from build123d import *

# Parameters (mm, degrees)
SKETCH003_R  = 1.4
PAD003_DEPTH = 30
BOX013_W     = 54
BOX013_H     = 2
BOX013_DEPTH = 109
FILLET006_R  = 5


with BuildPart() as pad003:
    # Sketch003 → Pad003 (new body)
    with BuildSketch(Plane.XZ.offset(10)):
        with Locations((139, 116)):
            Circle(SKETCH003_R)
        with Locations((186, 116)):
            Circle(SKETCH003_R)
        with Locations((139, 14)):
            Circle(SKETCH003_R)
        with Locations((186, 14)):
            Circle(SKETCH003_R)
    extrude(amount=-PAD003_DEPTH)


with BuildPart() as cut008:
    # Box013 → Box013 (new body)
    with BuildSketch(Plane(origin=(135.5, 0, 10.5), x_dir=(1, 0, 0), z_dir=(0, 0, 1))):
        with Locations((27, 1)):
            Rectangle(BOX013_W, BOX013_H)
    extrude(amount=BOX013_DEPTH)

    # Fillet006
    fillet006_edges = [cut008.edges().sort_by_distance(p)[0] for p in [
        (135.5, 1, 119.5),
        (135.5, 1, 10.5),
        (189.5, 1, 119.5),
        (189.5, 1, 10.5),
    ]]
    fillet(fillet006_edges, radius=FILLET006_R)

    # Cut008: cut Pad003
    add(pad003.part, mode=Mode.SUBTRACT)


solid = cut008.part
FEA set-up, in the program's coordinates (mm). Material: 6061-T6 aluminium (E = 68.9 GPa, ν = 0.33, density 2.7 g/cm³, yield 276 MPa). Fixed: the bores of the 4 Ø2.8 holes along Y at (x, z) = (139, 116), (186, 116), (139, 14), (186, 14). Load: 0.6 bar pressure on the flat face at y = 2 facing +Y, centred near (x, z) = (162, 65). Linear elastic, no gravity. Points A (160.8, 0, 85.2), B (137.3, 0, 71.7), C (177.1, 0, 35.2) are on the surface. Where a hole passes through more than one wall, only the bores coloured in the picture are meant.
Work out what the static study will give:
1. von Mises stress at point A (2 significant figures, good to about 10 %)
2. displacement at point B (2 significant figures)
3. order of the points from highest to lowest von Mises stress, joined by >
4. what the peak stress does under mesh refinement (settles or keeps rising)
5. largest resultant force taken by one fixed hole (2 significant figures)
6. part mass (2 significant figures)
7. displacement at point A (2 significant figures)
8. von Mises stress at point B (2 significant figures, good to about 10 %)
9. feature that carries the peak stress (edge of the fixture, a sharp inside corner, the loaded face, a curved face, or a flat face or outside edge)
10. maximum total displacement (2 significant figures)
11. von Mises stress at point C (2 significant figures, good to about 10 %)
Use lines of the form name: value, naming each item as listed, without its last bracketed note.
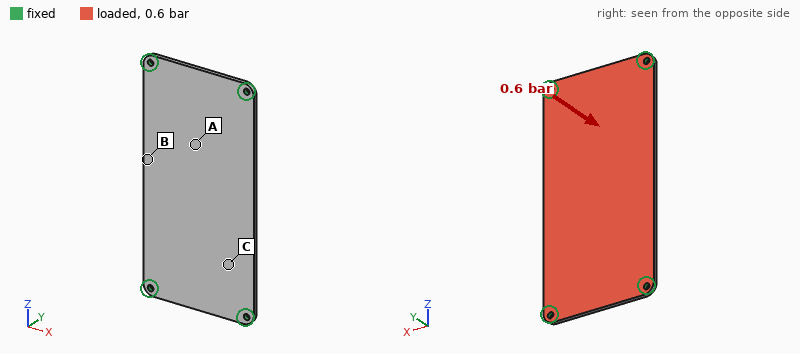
von Mises stress at point A: 25 MPa
displacement at point B: 0.50 mm
order of the points from highest to lowest von Mises stress, joined by >: B > A > C
what the peak stress does under mesh refinement: keeps rising
largest resultant force taken by one fixed hole: 88 N
part mass: 32 g
displacement at point A: 0.38 mm
von Mises stress at point B: 48 MPa
feature that carries the peak stress: edge of the fixture
maximum total displacement: 0.52 mm
von Mises stress at point C: 15 MPa
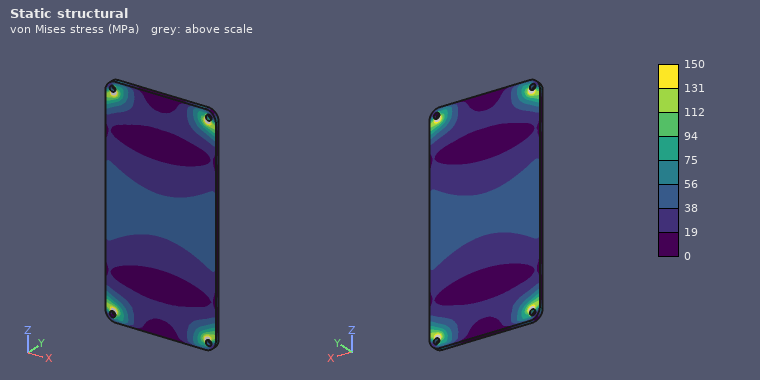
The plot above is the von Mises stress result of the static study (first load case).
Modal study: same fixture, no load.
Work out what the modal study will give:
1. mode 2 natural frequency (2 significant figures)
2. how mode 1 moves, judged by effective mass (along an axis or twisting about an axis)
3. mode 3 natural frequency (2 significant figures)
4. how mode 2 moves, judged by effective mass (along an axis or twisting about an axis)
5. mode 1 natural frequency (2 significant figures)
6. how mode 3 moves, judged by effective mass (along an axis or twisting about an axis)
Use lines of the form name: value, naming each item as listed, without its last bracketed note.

mode 2 natural frequency: 1600 Hz
how mode 1 moves, judged by effective mass: along Y
mode 3 natural frequency: 2400 Hz
how mode 2 moves, judged by effective mass: twisting about Z
mode 1 natural frequency: 850 Hz
how mode 3 moves, judged by effective mass: twisting about X
